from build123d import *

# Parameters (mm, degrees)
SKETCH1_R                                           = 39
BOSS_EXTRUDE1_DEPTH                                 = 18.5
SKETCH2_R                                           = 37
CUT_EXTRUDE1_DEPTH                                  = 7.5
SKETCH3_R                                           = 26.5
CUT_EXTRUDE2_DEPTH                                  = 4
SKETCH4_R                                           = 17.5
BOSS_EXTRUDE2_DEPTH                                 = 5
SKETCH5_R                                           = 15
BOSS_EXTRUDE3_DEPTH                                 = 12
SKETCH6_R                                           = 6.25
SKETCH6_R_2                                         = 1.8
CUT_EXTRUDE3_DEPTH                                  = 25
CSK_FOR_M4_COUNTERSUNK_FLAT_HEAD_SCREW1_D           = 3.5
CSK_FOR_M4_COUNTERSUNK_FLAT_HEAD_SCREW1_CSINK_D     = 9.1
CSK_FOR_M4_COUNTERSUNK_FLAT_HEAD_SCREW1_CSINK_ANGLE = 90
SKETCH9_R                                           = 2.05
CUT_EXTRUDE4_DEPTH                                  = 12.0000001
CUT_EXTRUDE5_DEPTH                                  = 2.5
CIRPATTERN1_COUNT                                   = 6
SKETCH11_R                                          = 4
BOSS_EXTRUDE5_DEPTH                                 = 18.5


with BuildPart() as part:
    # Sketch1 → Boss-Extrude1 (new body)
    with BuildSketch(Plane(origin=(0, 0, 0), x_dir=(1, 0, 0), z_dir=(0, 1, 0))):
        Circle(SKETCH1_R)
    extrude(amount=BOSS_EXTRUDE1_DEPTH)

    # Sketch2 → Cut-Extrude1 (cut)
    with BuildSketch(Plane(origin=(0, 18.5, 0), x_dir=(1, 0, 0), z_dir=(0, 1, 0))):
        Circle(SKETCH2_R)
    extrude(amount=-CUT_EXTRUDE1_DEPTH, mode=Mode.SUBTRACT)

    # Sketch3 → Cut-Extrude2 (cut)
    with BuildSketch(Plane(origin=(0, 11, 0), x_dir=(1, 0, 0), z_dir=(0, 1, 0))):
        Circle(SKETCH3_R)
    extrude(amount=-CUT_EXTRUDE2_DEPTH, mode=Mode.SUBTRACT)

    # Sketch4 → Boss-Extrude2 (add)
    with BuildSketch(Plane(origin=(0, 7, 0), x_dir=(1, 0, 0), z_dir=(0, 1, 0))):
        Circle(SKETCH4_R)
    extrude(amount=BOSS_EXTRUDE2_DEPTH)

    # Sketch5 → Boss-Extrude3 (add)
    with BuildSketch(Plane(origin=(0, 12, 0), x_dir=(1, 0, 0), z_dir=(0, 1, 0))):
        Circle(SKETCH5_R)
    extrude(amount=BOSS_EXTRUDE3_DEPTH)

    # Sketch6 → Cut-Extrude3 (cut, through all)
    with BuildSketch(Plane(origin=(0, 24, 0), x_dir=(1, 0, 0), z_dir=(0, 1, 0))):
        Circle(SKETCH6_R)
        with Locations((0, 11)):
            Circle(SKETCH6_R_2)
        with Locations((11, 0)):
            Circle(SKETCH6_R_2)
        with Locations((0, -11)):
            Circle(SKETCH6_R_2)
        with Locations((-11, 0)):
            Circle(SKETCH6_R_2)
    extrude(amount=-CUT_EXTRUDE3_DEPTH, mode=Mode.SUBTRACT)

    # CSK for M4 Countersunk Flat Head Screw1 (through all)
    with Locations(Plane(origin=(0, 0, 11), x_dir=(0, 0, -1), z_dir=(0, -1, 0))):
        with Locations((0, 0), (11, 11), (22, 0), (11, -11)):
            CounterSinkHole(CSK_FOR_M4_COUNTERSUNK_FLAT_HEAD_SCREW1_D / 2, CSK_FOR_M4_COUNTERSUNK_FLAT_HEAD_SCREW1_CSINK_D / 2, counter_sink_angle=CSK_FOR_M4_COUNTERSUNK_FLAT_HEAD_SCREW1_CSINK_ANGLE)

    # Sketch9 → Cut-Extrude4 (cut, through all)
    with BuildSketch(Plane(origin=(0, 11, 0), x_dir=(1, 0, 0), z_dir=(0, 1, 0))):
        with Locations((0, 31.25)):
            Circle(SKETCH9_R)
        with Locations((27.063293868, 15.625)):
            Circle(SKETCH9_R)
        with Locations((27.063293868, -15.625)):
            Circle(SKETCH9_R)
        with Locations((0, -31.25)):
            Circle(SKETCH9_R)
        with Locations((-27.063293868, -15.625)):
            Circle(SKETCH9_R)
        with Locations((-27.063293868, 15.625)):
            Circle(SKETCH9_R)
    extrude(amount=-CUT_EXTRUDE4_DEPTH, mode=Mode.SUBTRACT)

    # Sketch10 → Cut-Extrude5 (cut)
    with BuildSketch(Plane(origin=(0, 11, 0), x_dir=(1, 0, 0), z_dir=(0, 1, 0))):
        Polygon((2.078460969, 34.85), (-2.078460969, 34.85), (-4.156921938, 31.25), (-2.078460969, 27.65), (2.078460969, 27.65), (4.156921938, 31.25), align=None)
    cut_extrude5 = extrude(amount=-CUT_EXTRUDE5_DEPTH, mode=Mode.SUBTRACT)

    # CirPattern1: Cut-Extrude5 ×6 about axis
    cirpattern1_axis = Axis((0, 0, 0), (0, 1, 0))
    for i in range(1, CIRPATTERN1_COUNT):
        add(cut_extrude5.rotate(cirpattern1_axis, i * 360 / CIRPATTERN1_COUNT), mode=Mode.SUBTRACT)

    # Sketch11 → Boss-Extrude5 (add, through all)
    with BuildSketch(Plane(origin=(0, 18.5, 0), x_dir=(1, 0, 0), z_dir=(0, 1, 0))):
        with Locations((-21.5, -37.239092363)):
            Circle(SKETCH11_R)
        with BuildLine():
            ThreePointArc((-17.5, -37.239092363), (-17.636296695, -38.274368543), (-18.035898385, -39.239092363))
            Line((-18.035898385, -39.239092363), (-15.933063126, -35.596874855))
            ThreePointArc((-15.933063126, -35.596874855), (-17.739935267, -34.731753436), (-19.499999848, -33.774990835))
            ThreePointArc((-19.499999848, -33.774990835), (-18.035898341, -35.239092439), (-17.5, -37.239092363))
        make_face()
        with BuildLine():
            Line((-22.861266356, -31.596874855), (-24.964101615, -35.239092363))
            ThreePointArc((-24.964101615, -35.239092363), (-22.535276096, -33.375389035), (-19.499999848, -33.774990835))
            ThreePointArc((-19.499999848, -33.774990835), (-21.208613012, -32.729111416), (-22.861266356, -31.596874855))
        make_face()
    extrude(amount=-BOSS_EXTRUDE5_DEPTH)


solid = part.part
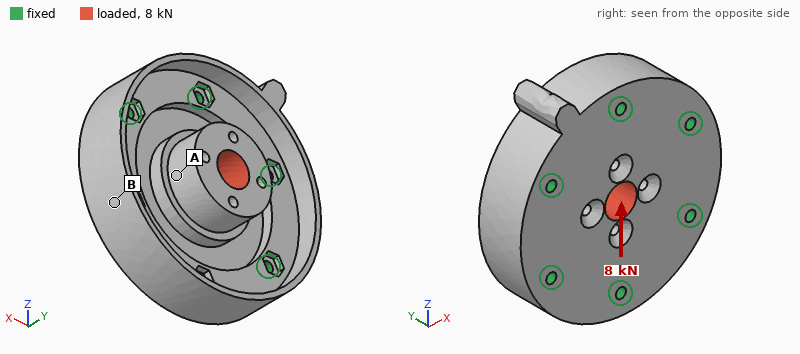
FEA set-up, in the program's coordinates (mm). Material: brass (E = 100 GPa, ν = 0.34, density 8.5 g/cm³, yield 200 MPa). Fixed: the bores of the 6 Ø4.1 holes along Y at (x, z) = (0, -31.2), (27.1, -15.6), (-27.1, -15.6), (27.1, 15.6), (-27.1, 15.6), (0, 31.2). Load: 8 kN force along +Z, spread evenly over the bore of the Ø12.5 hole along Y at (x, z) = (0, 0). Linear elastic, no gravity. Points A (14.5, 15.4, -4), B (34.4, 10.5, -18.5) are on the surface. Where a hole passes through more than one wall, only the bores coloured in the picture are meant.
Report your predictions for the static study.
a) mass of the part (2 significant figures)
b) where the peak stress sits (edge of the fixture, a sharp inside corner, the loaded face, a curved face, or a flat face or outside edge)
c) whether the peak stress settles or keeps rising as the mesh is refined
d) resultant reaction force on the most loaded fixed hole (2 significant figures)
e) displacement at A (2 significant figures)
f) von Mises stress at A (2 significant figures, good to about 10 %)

480 g
edge of the fixture
keeps rising
2.2 kN
8.1 µm
11 MPa
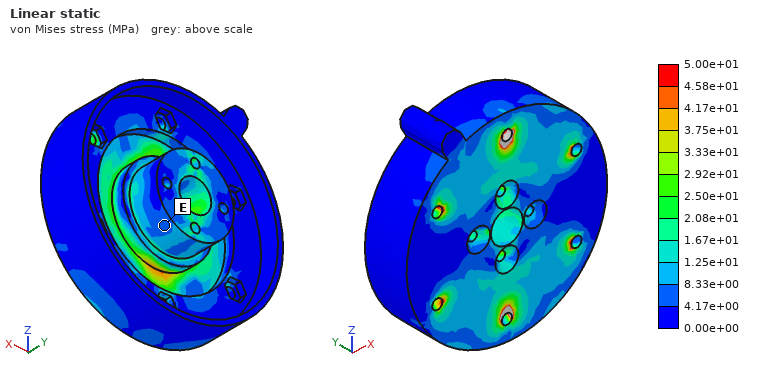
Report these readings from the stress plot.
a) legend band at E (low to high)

4.17e+00 to 8.33e+00 MPa
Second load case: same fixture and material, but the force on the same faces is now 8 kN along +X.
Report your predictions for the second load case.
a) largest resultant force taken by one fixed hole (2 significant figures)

1.9 kN
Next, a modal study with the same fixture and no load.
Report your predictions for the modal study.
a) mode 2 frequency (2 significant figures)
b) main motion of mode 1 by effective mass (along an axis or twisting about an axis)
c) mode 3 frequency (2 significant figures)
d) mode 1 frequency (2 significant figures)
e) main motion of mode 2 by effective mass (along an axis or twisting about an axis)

10 kHz
along Y
12 kHz
9200 Hz
along Y
